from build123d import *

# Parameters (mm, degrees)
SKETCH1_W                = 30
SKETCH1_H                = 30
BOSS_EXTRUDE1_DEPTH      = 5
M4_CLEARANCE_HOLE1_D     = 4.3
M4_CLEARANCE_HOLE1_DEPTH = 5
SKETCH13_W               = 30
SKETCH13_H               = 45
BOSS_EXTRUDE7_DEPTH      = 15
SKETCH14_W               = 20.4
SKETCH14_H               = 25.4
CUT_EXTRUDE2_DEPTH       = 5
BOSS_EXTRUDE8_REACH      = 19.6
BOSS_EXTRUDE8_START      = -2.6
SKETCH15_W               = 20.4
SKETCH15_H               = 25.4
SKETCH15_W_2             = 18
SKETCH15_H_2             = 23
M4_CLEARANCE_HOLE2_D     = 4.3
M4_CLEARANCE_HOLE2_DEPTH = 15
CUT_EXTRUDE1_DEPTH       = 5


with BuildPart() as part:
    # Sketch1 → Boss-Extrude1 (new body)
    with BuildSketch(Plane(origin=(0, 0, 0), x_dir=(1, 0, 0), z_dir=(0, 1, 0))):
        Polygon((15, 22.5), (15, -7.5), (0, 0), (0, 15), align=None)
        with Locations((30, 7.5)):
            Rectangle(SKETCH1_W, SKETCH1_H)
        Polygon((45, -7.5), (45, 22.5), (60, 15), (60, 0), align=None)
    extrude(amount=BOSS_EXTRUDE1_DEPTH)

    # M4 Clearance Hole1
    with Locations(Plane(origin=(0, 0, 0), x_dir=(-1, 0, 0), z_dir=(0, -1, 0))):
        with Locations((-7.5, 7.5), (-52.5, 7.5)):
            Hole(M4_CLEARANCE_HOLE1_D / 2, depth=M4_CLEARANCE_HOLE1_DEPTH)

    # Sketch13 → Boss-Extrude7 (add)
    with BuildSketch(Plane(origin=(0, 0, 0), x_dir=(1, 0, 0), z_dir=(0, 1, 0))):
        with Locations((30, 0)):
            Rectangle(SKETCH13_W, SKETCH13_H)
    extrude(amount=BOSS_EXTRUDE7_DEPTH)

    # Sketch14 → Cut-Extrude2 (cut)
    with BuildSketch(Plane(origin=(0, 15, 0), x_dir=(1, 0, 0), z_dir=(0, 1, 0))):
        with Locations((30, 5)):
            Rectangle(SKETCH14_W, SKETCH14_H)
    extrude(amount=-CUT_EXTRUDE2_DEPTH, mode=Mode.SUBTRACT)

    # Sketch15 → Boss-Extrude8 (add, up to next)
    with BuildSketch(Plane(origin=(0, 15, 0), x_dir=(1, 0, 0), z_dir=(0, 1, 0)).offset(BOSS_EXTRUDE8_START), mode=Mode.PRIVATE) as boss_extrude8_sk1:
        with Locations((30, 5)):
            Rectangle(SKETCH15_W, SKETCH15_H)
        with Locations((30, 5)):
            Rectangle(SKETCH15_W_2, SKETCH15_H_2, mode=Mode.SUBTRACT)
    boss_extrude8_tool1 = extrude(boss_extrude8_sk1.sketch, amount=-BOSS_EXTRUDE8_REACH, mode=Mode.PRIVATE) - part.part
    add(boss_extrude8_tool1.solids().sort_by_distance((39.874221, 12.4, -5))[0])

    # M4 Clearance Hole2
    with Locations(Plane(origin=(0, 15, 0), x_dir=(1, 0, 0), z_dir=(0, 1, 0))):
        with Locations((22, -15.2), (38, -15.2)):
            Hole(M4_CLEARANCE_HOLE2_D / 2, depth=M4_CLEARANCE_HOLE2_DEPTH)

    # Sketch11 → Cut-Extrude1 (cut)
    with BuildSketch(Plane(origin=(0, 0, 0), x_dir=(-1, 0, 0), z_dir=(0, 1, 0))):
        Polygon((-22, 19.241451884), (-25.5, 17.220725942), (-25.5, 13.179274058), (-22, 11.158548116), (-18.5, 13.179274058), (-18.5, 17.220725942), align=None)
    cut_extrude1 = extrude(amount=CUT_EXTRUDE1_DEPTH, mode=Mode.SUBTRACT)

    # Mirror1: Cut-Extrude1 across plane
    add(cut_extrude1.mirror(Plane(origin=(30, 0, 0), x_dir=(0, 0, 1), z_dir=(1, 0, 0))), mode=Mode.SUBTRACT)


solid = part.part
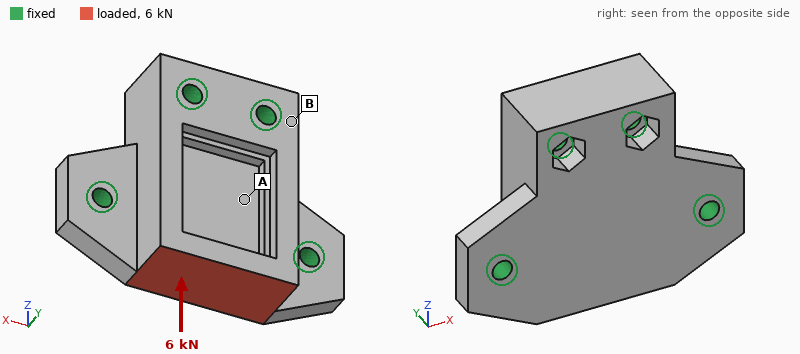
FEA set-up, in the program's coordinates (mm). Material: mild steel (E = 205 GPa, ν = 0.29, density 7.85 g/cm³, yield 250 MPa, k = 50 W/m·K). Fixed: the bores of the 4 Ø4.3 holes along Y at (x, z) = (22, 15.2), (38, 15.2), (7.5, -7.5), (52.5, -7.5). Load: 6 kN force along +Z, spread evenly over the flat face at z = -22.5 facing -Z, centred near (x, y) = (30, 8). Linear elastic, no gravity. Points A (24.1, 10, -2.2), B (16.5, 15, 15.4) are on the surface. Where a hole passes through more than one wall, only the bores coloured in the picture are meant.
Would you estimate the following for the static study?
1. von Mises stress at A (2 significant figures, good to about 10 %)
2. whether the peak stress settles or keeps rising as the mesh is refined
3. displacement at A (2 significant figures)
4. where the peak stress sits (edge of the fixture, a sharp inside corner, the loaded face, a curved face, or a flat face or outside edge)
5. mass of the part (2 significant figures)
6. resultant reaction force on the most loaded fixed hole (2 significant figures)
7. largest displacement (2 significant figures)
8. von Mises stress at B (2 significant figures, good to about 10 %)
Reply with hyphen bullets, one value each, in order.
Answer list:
- 25 MPa
- keeps rising
- 1.8 µm
- edge of the fixture
- 160 g
- 2.2 kN
- 8.6 µm
- 8.2 MPa
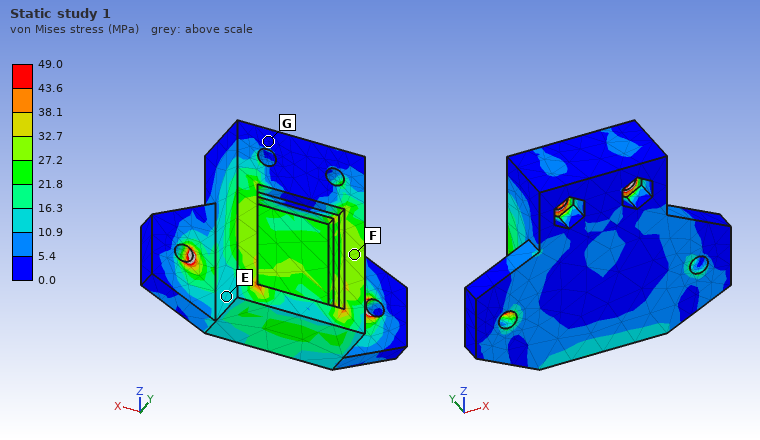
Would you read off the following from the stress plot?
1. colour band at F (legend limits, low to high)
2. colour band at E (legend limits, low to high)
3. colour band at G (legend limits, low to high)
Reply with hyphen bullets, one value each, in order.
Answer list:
- 27.2 to 32.7 MPa
- 10.9 to 16.3 MPa
- 0.0 to 5.4 MPa
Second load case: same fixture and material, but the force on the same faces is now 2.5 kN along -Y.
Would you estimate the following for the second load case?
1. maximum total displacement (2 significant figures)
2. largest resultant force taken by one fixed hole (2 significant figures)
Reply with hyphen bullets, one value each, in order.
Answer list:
- 18 µm
- 1.8 kN
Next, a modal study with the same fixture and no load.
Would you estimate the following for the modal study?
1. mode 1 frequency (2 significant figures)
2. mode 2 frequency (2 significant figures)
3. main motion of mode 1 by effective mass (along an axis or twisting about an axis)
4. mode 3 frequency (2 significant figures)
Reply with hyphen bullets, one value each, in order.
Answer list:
- 12 kHz
- 23 kHz
- along Y
- 28 kHz
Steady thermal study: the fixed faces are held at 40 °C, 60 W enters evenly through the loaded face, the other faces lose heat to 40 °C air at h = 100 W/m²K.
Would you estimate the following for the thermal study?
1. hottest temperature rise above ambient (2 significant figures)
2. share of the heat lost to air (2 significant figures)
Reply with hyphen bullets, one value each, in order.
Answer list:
- 73 K
- 20 %
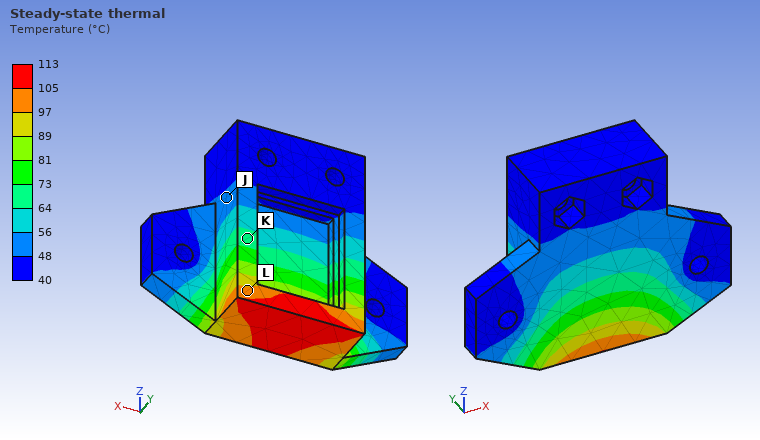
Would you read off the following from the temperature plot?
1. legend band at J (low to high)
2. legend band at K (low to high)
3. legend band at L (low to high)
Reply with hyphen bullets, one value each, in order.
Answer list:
- 48 to 56 °C
- 64 to 73 °C
- 97 to 105 °C
